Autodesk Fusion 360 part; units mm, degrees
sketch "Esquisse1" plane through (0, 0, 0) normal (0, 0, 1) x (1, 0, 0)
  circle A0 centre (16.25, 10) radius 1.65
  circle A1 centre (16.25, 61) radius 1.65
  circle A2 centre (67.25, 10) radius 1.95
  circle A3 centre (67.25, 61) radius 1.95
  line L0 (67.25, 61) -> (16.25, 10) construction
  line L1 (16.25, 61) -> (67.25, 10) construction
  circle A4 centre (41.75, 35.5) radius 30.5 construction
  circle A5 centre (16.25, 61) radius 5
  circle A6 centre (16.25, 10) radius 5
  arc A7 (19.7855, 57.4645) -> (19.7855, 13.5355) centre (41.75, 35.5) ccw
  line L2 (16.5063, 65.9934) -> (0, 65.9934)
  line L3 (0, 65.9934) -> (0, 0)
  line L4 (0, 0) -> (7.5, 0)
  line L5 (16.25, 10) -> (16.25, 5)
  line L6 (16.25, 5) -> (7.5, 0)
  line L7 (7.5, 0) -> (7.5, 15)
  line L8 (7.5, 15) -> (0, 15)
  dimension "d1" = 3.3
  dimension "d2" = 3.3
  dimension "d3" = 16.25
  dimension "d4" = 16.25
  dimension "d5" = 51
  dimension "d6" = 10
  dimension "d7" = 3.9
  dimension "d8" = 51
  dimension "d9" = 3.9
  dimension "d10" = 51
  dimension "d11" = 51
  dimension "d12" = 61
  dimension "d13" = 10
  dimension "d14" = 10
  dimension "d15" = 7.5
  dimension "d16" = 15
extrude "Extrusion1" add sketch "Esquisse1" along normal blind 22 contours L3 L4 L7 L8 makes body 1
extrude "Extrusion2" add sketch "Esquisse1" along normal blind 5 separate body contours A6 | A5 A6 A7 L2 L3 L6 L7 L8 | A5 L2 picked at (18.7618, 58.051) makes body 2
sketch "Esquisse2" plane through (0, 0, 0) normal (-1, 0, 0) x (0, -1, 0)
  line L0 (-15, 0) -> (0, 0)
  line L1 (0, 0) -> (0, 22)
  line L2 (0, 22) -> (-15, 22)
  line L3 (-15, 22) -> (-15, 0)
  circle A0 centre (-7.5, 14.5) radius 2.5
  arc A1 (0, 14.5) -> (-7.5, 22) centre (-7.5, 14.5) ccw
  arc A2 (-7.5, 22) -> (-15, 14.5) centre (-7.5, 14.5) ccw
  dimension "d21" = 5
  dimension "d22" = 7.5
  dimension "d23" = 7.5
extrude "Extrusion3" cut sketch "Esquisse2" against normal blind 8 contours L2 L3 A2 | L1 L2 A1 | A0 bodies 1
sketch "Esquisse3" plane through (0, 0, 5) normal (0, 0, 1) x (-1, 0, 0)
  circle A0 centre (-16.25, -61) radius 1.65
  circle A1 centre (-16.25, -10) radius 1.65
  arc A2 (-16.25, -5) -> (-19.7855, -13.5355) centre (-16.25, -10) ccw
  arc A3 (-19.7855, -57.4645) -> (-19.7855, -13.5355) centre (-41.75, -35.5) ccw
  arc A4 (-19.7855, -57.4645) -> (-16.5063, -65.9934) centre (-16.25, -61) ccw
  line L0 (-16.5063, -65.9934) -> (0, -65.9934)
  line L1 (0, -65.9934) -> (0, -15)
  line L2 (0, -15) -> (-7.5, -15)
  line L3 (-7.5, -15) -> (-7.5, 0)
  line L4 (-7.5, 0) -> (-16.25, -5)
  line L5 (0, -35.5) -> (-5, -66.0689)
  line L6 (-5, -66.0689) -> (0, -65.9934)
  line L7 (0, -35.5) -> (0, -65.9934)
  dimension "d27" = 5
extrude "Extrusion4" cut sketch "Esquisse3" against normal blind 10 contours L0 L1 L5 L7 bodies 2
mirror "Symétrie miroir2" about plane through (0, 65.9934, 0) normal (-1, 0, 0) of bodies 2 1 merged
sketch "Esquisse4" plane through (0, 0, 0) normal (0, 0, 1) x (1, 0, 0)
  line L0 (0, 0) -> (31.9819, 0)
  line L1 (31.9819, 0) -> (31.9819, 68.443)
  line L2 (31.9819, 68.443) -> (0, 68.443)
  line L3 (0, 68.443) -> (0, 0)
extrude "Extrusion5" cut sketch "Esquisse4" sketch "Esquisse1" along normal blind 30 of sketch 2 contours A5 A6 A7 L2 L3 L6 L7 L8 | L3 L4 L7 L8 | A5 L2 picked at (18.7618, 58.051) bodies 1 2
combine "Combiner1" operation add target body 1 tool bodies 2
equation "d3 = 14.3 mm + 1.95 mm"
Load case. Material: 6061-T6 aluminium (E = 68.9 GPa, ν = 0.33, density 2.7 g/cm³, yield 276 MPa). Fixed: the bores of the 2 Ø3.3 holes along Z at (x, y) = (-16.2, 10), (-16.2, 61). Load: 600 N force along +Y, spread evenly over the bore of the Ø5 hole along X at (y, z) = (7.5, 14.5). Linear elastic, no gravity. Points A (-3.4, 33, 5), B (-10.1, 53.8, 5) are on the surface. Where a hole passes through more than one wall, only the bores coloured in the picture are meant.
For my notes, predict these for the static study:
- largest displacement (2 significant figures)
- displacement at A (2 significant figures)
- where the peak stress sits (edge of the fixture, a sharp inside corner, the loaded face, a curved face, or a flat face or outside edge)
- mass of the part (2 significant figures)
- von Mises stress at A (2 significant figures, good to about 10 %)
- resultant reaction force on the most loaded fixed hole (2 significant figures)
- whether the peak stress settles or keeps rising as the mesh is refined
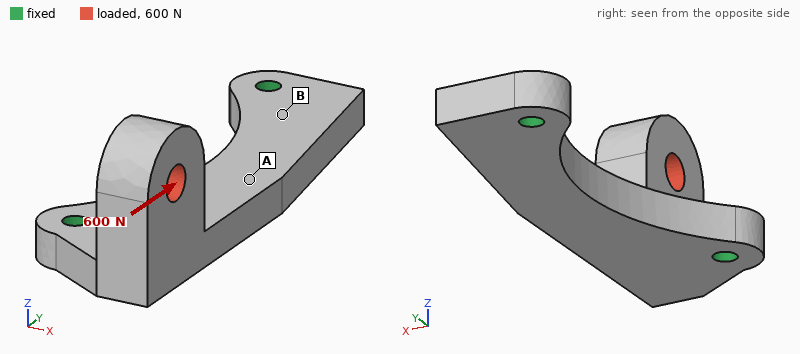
83 µm
30 µm
edge of the fixture
17 g
24 MPa
340 N
keeps rising
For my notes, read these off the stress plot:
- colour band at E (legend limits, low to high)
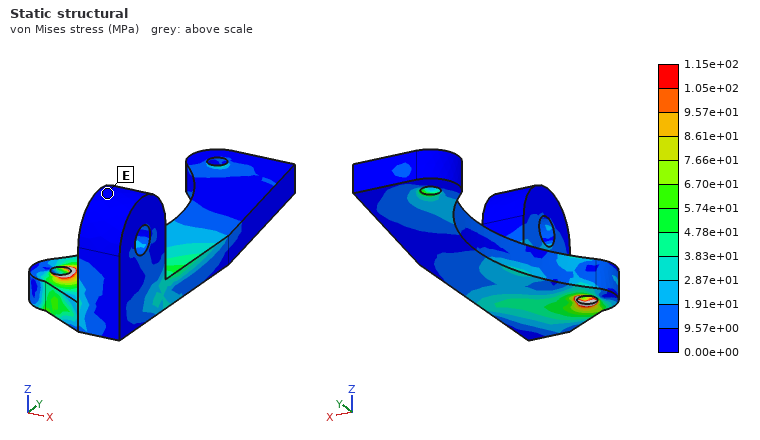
0.00e+00 to 9.57e+00 MPa
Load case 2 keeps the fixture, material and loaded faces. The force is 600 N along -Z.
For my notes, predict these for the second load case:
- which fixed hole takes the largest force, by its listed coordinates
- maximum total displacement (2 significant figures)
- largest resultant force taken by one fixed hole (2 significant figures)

(-16.2, 10)
100 µm
600 N
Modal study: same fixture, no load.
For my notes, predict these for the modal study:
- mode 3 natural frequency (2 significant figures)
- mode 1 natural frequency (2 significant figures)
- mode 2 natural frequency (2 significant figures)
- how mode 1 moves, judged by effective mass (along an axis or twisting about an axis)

11 kHz
5000 Hz
6600 Hz
along Z
